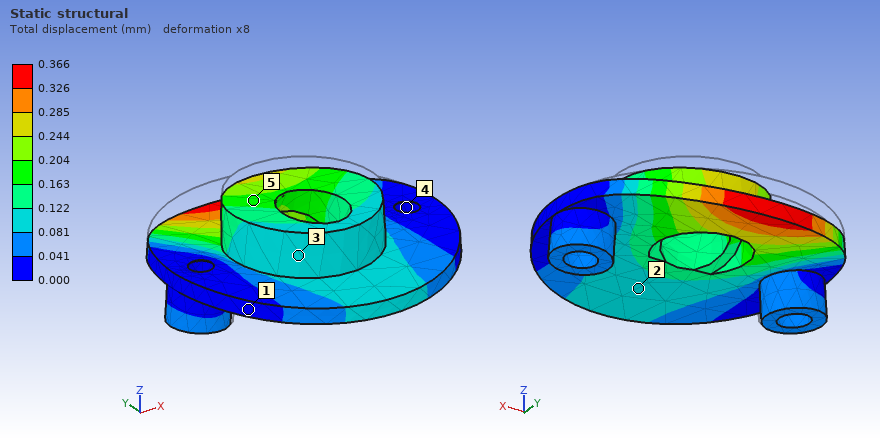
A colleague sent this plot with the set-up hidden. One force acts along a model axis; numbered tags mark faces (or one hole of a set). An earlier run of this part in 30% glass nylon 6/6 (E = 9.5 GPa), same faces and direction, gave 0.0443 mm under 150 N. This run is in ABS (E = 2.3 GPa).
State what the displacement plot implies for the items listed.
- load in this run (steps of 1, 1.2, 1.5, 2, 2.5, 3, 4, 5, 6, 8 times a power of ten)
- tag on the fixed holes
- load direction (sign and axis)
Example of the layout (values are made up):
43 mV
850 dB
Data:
300 N
4
-Z
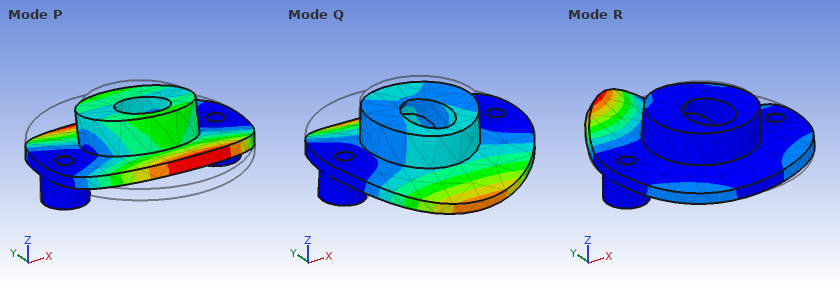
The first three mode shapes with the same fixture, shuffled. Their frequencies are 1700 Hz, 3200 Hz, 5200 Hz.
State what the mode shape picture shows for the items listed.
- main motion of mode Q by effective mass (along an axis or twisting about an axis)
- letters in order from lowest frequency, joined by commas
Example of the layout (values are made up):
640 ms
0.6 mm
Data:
along Z
P, Q, R
